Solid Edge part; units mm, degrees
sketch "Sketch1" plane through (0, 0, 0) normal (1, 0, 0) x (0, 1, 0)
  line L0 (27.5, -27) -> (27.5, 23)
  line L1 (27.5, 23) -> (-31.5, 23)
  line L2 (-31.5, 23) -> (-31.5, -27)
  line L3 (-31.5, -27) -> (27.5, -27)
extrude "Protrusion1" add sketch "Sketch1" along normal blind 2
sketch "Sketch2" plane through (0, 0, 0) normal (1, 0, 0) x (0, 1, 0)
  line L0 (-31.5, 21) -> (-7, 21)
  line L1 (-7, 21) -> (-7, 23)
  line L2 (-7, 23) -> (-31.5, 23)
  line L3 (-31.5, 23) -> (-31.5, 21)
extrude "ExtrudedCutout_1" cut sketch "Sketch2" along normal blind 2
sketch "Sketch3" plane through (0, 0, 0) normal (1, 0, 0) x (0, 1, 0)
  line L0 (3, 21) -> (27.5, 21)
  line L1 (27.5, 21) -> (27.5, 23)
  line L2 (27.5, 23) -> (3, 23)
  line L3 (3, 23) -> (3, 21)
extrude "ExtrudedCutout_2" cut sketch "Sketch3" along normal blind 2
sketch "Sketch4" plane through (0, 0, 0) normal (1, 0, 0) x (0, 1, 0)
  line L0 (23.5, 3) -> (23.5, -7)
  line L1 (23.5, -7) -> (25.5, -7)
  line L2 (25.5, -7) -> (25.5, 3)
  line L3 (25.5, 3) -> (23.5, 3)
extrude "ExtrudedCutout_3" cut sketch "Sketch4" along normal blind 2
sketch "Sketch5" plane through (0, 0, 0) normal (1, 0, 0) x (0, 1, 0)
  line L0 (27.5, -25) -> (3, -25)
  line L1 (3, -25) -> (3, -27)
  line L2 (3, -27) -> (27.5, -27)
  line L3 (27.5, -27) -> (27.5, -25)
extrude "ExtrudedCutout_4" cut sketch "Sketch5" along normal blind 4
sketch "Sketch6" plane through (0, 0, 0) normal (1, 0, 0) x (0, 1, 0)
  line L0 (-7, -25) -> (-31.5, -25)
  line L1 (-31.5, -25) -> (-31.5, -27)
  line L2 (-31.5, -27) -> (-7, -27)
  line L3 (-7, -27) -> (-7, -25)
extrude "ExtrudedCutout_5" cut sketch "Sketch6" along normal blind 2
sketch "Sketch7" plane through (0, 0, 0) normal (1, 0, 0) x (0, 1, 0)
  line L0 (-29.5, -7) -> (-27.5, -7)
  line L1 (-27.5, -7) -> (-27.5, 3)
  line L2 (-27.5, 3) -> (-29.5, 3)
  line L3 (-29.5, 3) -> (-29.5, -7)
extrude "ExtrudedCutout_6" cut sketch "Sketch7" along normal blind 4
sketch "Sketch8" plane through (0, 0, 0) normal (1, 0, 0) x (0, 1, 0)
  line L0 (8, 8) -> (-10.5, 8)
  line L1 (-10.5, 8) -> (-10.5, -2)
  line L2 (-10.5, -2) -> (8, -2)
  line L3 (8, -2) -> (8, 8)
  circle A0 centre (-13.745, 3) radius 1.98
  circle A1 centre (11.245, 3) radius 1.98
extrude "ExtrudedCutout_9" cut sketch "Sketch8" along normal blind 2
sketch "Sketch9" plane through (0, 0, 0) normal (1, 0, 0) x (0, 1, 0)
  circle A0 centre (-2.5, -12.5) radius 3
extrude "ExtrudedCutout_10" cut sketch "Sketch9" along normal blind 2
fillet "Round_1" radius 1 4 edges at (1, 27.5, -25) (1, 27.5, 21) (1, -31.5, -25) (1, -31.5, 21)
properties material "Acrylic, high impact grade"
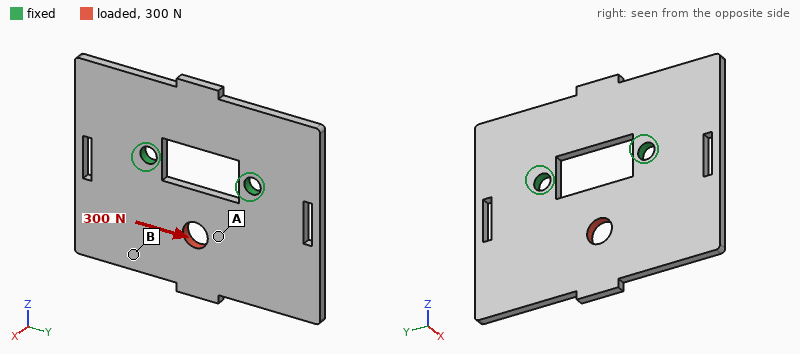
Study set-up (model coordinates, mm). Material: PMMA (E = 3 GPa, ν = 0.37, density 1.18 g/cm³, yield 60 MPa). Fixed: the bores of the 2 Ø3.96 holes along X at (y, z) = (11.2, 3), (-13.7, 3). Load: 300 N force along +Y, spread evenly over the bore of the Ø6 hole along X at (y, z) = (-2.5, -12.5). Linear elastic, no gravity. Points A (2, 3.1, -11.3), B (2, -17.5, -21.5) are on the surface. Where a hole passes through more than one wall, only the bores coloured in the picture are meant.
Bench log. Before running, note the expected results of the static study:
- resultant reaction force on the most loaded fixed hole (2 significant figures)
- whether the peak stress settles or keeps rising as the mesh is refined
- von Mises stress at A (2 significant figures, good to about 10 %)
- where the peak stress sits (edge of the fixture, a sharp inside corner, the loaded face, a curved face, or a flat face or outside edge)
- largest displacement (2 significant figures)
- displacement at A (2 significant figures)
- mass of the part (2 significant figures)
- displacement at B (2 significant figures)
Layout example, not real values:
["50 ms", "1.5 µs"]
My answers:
["210 N", "keeps rising", "11 MPa", "edge of the fixture", "0.19 mm", "0.11 mm", "5.8 g", "0.15 mm"]
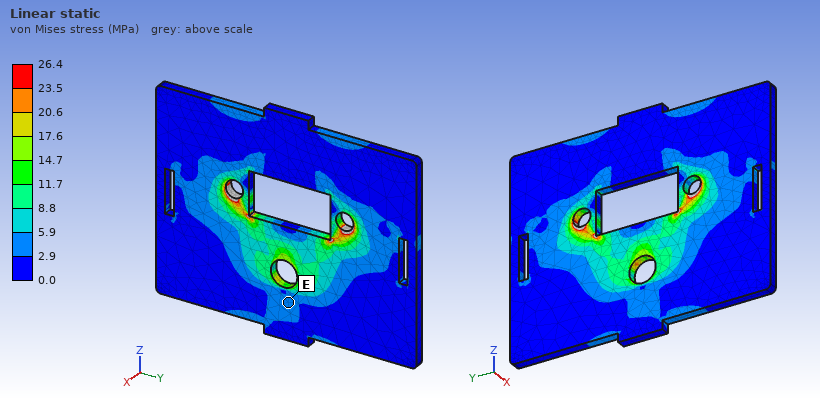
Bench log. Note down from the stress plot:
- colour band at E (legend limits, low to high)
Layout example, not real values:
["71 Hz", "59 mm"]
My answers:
["2.9 to 5.9 MPa"]
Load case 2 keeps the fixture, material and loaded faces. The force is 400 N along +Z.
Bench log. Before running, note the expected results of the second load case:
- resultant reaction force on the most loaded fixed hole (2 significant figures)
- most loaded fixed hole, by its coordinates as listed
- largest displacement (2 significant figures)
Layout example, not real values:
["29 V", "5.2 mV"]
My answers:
["230 N", "(-13.7, 3)", "0.10 mm"]
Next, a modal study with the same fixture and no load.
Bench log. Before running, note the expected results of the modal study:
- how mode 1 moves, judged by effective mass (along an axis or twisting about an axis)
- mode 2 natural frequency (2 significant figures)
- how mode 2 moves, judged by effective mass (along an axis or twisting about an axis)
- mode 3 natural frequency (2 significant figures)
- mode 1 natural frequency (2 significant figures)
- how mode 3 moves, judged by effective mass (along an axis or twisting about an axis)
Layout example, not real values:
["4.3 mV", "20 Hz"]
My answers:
["along X", "810 Hz", "twisting about Z", "1200 Hz", "530 Hz", "along X"]
